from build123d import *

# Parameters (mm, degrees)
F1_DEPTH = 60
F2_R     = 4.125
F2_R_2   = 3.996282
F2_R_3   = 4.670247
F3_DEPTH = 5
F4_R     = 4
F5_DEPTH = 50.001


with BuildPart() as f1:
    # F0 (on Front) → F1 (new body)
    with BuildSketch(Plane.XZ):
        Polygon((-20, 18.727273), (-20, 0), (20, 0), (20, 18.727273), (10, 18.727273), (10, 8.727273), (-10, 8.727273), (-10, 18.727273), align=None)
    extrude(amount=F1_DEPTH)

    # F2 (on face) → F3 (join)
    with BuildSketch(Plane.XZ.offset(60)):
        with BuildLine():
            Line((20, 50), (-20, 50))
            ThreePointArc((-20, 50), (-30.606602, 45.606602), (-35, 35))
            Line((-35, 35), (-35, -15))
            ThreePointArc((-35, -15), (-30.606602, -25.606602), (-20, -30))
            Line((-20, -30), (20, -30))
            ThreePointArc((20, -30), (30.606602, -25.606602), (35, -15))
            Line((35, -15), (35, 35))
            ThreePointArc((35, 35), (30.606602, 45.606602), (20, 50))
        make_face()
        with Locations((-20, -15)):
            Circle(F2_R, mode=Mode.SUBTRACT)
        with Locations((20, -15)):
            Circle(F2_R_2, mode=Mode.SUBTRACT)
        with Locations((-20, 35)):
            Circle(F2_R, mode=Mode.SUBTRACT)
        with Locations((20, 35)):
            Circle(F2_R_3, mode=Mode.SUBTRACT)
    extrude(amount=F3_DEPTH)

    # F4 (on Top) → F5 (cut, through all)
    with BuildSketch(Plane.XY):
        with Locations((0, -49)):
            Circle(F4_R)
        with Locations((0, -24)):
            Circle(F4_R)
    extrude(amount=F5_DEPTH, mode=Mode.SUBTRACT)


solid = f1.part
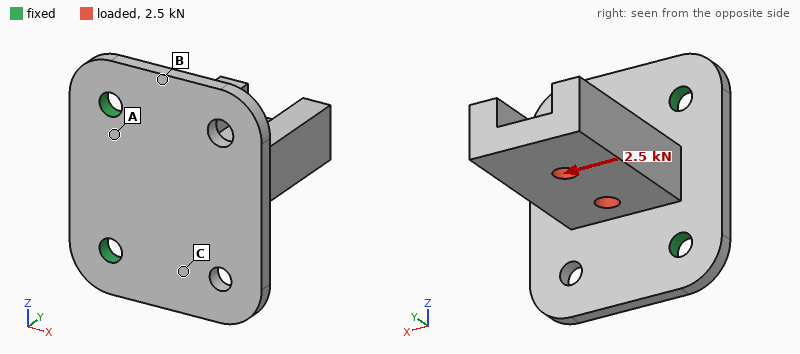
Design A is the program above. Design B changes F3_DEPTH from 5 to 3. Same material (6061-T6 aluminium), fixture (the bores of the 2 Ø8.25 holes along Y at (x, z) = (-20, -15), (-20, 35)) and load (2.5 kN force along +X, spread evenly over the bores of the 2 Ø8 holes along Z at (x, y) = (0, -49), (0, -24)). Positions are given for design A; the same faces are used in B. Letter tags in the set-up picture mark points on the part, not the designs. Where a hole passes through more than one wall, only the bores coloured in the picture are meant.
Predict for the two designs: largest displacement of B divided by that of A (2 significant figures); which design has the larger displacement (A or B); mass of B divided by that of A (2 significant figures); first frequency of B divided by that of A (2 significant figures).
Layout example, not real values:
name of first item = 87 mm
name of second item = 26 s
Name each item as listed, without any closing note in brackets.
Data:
largest displacement of B divided by that of A = 3.5
which design has the larger displacement = B
mass of B divided by that of A = 0.82
first frequency of B divided by that of A = 0.55
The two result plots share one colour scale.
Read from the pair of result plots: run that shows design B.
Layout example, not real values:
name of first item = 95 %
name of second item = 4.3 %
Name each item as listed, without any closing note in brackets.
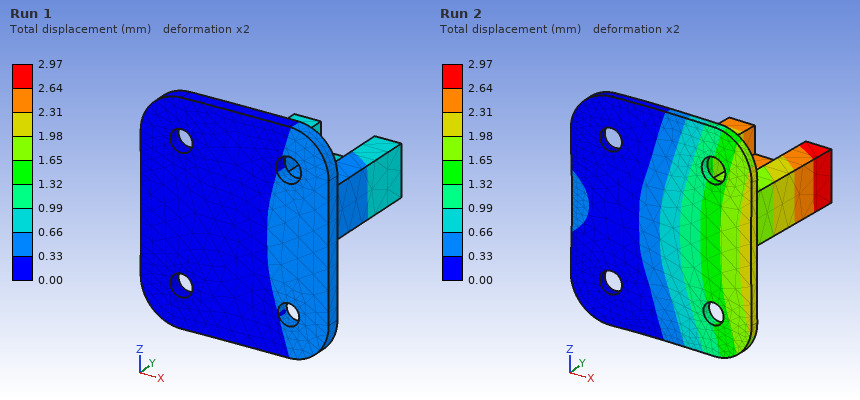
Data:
run that shows design B = Run 2
